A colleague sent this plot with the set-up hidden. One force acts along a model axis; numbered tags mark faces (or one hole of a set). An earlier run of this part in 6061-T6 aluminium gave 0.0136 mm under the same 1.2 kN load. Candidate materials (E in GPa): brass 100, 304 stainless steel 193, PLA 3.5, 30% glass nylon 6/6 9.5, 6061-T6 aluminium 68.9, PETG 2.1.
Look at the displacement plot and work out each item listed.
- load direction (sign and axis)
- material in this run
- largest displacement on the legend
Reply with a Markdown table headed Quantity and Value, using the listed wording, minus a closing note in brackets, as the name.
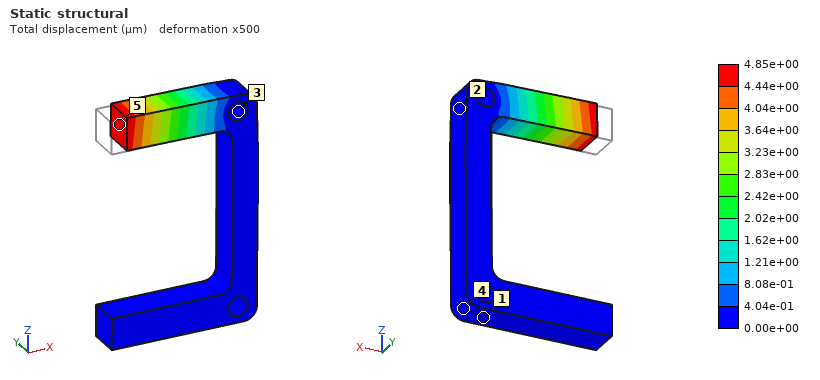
| Quantity | Value |
|---|---|
| load direction | +X |
| material in this run | 304 stainless steel |
| largest displacement on the legend | 4.85e+00 µm |
